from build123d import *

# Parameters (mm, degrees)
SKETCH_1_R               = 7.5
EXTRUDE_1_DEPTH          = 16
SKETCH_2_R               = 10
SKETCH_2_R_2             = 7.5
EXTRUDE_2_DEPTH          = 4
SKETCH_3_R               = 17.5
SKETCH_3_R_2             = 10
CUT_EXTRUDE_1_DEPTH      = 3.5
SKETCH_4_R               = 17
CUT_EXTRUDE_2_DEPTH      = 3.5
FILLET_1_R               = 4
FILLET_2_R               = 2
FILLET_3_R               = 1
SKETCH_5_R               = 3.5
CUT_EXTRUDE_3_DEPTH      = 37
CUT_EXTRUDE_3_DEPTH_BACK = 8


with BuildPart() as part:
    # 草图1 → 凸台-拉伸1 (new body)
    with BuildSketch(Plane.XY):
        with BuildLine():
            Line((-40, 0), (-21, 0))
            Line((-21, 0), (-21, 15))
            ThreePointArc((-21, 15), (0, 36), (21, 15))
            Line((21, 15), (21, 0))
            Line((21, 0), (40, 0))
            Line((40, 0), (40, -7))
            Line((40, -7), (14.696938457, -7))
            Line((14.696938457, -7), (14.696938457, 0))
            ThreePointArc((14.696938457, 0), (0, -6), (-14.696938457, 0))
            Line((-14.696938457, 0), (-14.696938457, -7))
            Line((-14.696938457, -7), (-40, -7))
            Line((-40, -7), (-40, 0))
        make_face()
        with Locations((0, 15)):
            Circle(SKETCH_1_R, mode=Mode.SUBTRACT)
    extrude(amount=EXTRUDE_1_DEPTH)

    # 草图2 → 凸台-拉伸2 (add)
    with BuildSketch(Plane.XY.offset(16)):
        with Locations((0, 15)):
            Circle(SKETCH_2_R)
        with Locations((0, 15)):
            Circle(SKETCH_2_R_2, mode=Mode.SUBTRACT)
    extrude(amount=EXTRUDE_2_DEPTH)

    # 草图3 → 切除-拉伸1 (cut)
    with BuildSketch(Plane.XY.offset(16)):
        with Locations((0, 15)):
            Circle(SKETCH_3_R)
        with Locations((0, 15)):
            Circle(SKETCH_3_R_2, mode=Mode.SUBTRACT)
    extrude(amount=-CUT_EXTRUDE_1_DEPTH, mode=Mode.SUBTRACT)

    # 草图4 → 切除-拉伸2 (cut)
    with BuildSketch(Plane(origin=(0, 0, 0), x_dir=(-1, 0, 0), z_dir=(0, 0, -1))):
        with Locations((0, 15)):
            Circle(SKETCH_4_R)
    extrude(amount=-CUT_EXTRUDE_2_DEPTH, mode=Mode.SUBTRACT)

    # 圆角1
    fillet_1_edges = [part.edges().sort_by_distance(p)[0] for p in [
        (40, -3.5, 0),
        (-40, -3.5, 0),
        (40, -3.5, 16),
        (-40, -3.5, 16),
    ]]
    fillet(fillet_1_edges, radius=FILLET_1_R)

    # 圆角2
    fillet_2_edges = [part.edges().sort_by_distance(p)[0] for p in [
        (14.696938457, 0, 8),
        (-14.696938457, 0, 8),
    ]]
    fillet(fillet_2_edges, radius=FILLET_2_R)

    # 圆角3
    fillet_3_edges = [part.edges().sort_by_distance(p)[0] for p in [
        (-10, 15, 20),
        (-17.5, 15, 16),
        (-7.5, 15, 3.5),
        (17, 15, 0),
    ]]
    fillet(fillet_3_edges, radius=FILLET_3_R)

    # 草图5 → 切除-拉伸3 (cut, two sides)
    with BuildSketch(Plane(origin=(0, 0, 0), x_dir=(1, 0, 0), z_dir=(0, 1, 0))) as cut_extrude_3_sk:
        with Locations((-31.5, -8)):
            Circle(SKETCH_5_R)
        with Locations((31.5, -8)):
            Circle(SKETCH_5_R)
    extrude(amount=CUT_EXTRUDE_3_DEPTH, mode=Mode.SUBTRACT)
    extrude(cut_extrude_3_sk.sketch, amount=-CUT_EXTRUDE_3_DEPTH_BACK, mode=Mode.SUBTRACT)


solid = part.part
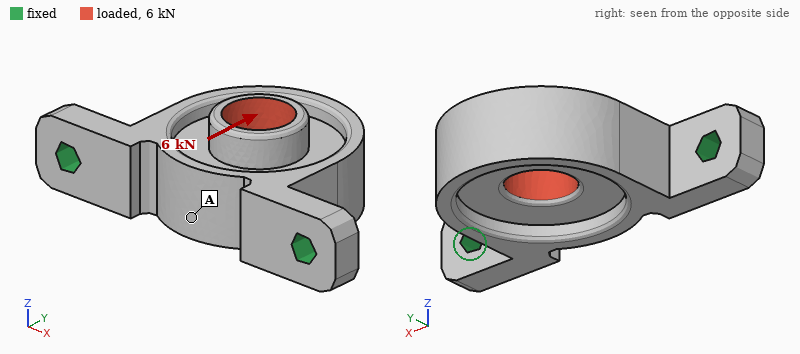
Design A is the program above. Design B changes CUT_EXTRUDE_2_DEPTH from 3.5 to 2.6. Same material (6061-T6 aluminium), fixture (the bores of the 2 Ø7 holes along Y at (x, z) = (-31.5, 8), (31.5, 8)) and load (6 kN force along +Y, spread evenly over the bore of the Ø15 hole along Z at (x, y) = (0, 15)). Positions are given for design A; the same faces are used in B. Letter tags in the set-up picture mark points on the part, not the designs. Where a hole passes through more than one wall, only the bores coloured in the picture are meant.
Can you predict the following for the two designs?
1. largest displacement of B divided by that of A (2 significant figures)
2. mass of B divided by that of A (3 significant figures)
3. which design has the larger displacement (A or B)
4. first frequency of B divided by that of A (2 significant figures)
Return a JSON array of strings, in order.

["0.91", "1.03", "A", "0.98"]
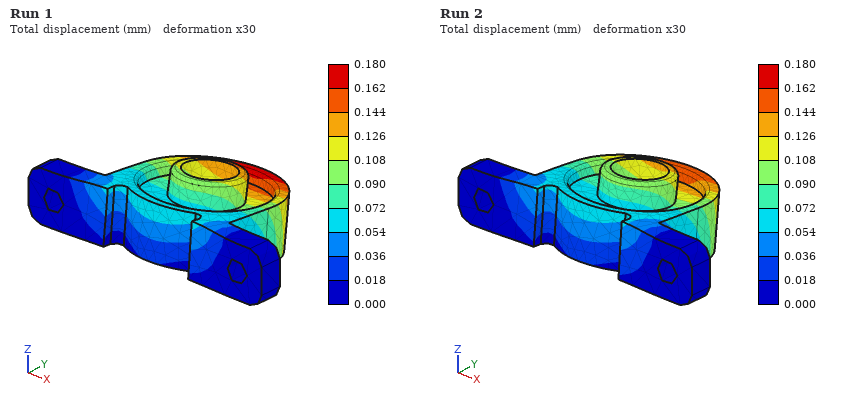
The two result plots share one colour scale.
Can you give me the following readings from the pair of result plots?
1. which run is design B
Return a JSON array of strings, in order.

["Run 2"]
